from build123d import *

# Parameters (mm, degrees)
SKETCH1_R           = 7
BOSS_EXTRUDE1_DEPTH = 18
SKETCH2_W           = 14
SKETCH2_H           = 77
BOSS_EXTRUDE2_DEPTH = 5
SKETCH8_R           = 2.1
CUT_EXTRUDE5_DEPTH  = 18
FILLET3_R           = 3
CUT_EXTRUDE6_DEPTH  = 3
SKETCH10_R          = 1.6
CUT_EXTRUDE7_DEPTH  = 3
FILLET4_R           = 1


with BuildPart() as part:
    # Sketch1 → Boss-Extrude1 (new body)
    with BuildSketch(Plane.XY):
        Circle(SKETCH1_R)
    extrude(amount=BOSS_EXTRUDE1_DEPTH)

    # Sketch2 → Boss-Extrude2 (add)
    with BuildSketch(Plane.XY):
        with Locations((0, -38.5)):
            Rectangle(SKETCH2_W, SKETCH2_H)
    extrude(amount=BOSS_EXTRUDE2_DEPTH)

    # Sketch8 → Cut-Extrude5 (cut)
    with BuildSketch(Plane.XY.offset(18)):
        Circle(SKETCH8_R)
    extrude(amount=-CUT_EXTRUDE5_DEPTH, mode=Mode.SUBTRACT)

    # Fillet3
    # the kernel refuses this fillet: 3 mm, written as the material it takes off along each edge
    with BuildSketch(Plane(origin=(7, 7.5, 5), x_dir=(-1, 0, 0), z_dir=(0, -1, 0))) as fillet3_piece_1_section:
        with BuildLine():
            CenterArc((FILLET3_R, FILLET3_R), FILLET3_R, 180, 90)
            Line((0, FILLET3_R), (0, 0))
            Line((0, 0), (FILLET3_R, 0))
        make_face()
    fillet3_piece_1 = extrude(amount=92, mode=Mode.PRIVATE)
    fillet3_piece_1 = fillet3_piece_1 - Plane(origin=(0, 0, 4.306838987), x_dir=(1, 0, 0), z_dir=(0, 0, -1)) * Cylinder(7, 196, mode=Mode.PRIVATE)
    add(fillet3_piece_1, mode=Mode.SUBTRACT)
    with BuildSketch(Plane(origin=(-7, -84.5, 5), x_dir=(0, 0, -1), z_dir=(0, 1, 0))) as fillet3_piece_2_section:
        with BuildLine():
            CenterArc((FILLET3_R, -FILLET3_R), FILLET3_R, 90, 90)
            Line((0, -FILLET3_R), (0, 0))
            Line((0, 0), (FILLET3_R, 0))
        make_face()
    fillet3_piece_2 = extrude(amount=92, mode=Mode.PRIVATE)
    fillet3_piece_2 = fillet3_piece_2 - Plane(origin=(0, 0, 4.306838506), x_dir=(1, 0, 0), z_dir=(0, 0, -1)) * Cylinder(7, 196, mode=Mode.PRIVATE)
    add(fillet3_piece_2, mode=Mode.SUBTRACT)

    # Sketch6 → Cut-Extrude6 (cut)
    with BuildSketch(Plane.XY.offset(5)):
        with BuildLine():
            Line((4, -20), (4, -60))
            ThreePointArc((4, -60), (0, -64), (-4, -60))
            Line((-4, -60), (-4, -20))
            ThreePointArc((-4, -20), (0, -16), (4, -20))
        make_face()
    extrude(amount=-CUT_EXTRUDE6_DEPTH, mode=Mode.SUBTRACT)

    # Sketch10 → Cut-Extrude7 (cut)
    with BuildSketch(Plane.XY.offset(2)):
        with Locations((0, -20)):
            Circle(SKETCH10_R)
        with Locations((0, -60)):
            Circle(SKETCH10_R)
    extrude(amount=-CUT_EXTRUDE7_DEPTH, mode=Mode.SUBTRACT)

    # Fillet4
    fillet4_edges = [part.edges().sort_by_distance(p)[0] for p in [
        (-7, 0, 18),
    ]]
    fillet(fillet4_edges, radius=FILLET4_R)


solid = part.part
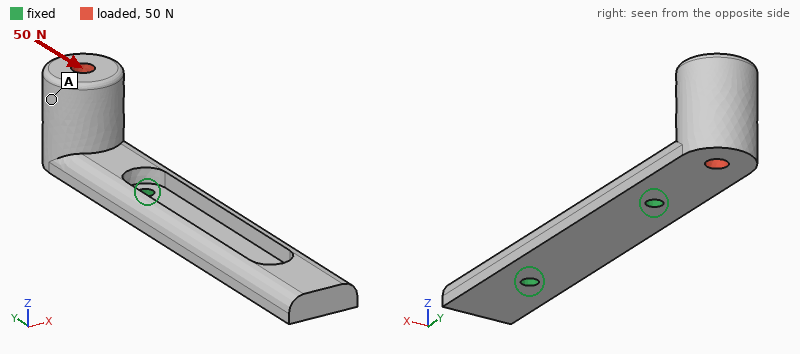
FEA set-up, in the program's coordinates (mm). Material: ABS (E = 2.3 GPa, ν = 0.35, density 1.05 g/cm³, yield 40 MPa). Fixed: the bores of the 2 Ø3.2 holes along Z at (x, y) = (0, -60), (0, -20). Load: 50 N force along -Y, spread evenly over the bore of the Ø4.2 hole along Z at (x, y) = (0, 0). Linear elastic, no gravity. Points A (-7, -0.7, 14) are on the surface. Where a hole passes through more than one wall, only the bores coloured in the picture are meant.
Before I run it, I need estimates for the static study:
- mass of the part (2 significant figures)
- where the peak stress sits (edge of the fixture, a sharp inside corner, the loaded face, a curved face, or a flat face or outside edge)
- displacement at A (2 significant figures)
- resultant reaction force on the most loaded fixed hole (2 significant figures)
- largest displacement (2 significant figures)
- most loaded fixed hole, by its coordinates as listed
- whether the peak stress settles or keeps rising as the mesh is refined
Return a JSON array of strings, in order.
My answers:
["6.4 g", "edge of the fixture", "0.61 mm", "27 N", "0.88 mm", "(0, -60)", "keeps rising"]
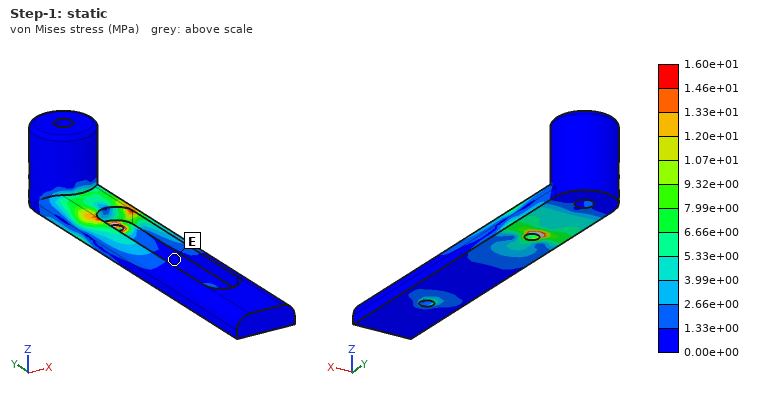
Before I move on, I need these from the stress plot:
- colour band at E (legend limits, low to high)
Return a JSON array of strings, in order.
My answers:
["0.00e+00 to 1.33e+00 MPa"]
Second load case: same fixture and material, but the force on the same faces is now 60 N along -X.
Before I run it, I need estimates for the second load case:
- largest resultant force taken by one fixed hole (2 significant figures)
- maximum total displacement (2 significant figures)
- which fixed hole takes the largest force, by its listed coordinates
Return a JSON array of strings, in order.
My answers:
["82 N", "0.87 mm", "(0, -20)"]
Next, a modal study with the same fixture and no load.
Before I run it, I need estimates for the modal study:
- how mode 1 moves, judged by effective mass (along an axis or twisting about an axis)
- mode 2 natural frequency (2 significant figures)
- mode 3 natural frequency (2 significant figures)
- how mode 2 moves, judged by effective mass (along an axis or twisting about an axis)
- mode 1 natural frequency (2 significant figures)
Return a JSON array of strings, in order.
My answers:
["along Z", "950 Hz", "2100 Hz", "along X", "560 Hz"]
